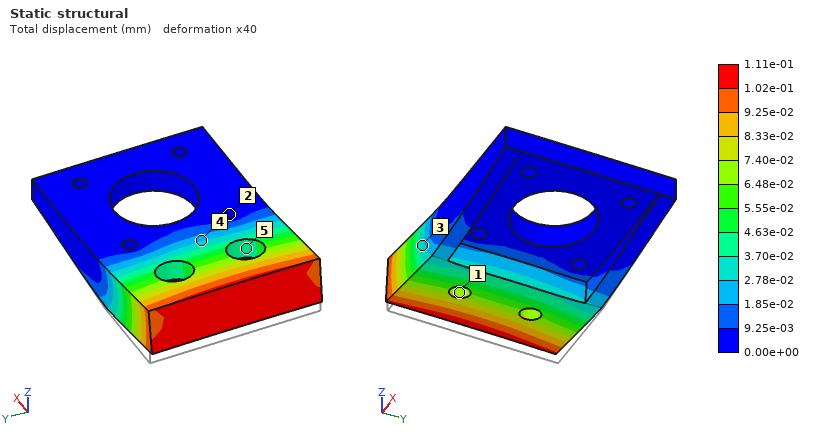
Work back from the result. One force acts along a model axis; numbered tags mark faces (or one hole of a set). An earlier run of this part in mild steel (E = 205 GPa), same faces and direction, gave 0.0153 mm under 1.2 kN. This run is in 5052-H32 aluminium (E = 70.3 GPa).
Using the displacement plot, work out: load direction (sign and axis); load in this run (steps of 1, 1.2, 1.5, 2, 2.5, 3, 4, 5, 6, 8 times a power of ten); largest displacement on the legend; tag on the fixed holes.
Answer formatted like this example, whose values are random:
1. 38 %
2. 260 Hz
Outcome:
1. +Z
2. 3 kN
3. 1.11e-01 mm
4. 2
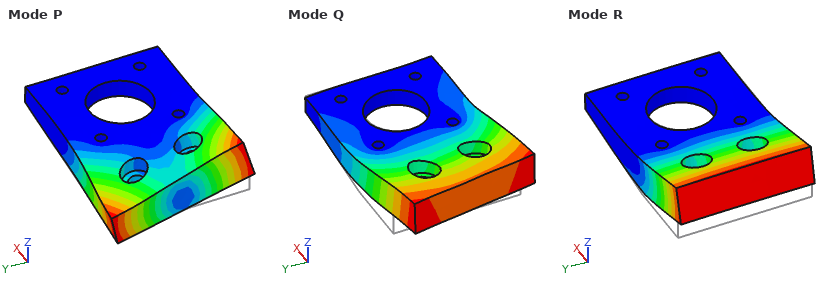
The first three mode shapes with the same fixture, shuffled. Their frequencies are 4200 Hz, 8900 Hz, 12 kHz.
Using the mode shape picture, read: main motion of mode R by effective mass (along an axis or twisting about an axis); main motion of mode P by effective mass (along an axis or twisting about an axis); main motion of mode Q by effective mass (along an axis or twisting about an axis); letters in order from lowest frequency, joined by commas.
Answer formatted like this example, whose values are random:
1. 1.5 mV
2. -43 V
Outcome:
1. along Z
2. twisting about X
3. along Y
4. R, P, Q
